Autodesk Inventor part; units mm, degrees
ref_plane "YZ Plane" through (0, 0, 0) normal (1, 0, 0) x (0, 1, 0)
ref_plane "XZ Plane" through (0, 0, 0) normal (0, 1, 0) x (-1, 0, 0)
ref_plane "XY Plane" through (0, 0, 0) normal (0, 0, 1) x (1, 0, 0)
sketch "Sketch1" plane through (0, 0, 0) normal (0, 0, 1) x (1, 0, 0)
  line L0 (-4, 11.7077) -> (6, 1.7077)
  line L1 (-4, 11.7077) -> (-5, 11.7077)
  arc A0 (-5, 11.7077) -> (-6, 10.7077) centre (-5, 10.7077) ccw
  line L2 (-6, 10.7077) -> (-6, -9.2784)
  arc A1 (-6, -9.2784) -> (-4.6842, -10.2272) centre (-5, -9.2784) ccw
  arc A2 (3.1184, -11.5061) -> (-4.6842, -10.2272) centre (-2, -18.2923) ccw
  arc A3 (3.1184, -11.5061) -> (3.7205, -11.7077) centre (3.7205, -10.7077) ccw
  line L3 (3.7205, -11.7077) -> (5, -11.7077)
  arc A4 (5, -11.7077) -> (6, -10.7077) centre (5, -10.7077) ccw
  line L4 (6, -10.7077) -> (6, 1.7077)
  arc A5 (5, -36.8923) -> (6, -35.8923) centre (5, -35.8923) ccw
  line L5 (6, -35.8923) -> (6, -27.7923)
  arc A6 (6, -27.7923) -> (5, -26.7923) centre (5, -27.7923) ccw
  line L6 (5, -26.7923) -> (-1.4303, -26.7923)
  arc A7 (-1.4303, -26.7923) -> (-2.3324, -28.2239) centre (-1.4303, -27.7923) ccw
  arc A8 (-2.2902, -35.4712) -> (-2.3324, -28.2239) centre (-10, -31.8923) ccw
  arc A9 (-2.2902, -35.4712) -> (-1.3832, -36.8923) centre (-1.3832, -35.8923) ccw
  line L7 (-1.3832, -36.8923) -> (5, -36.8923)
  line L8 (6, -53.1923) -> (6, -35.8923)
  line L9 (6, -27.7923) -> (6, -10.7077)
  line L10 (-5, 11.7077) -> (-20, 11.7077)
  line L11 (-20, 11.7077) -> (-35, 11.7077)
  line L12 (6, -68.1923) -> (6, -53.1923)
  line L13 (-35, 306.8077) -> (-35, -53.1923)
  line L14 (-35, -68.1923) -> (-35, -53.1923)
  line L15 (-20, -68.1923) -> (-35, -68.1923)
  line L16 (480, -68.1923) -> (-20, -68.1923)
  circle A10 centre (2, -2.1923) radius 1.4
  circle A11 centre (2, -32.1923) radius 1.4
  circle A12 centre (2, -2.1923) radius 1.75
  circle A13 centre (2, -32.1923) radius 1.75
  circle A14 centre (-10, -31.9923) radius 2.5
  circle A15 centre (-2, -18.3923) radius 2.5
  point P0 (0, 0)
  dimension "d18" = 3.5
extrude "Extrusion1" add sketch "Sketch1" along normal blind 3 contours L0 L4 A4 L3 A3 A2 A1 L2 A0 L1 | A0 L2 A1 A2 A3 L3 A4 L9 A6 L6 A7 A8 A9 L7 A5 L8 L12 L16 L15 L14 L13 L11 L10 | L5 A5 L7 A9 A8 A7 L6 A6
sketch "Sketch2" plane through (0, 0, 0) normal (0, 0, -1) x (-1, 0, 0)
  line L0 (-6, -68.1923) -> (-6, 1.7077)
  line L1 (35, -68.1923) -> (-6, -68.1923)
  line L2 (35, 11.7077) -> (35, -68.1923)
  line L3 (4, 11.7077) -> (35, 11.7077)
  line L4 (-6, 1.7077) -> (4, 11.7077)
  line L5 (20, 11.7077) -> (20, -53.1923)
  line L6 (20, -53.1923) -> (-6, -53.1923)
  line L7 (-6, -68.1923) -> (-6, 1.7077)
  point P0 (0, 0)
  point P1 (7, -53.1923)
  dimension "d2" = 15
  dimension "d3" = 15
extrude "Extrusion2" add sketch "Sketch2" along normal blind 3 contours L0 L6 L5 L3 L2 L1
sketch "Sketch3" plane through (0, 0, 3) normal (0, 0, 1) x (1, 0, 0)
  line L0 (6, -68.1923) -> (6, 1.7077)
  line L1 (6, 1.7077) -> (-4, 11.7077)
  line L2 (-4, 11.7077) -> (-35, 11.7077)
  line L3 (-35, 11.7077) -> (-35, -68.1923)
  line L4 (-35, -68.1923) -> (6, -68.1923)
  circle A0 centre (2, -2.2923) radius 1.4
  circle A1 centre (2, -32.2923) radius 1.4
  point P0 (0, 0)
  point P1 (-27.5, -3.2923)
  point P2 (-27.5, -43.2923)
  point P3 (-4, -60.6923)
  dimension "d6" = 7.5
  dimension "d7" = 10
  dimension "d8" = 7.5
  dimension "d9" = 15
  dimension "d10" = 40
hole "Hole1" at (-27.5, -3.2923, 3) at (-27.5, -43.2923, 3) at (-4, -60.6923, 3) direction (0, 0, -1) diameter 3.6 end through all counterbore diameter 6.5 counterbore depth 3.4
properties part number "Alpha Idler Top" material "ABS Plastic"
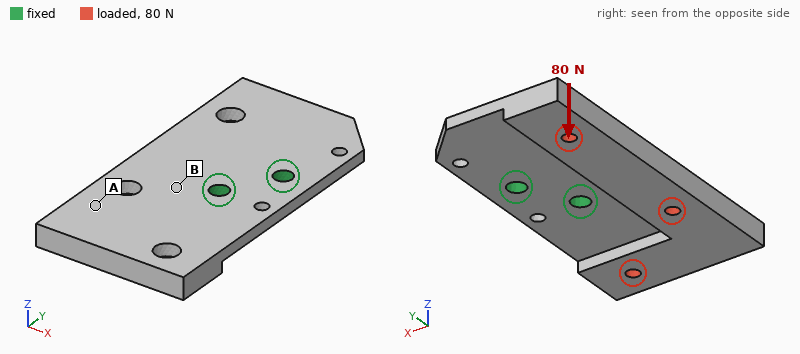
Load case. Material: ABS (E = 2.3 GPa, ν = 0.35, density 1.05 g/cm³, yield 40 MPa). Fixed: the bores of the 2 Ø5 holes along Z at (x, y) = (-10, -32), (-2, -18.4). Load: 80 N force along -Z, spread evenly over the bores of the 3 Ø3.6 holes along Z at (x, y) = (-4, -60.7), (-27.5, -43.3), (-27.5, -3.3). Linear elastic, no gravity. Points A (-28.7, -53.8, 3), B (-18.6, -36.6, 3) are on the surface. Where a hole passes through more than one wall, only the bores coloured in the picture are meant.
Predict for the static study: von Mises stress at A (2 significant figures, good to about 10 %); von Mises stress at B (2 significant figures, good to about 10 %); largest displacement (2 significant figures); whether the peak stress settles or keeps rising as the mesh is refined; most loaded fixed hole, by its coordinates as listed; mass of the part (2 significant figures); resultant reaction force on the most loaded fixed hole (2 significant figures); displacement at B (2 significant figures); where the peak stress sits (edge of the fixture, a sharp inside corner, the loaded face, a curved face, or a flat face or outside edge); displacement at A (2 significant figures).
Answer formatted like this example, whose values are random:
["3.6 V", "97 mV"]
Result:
["3.1 MPa", "7.4 MPa", "0.90 mm", "keeps rising", "(-10, -32)", "15 g", "89 N", "0.15 mm", "edge of the fixture", "0.58 mm"]
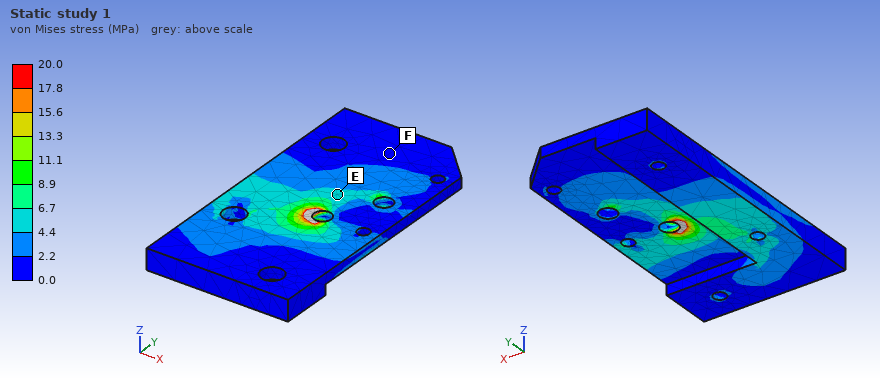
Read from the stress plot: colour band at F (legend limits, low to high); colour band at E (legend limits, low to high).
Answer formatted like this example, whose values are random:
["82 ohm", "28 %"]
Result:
["0.0 to 2.2 MPa", "4.4 to 6.7 MPa"]
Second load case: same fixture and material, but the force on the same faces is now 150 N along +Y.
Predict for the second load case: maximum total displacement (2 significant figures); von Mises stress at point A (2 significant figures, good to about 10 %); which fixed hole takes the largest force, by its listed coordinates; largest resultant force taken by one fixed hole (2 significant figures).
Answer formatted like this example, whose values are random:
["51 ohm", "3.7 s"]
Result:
["0.41 mm", "0.92 MPa", "(-10, -32)", "170 N"]
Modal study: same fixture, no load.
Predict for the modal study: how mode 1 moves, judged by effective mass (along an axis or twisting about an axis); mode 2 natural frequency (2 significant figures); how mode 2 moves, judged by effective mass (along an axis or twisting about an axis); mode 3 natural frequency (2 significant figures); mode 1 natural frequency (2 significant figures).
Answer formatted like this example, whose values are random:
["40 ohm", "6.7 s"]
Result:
["twisting about X", "580 Hz", "along Z", "870 Hz", "460 Hz"]
